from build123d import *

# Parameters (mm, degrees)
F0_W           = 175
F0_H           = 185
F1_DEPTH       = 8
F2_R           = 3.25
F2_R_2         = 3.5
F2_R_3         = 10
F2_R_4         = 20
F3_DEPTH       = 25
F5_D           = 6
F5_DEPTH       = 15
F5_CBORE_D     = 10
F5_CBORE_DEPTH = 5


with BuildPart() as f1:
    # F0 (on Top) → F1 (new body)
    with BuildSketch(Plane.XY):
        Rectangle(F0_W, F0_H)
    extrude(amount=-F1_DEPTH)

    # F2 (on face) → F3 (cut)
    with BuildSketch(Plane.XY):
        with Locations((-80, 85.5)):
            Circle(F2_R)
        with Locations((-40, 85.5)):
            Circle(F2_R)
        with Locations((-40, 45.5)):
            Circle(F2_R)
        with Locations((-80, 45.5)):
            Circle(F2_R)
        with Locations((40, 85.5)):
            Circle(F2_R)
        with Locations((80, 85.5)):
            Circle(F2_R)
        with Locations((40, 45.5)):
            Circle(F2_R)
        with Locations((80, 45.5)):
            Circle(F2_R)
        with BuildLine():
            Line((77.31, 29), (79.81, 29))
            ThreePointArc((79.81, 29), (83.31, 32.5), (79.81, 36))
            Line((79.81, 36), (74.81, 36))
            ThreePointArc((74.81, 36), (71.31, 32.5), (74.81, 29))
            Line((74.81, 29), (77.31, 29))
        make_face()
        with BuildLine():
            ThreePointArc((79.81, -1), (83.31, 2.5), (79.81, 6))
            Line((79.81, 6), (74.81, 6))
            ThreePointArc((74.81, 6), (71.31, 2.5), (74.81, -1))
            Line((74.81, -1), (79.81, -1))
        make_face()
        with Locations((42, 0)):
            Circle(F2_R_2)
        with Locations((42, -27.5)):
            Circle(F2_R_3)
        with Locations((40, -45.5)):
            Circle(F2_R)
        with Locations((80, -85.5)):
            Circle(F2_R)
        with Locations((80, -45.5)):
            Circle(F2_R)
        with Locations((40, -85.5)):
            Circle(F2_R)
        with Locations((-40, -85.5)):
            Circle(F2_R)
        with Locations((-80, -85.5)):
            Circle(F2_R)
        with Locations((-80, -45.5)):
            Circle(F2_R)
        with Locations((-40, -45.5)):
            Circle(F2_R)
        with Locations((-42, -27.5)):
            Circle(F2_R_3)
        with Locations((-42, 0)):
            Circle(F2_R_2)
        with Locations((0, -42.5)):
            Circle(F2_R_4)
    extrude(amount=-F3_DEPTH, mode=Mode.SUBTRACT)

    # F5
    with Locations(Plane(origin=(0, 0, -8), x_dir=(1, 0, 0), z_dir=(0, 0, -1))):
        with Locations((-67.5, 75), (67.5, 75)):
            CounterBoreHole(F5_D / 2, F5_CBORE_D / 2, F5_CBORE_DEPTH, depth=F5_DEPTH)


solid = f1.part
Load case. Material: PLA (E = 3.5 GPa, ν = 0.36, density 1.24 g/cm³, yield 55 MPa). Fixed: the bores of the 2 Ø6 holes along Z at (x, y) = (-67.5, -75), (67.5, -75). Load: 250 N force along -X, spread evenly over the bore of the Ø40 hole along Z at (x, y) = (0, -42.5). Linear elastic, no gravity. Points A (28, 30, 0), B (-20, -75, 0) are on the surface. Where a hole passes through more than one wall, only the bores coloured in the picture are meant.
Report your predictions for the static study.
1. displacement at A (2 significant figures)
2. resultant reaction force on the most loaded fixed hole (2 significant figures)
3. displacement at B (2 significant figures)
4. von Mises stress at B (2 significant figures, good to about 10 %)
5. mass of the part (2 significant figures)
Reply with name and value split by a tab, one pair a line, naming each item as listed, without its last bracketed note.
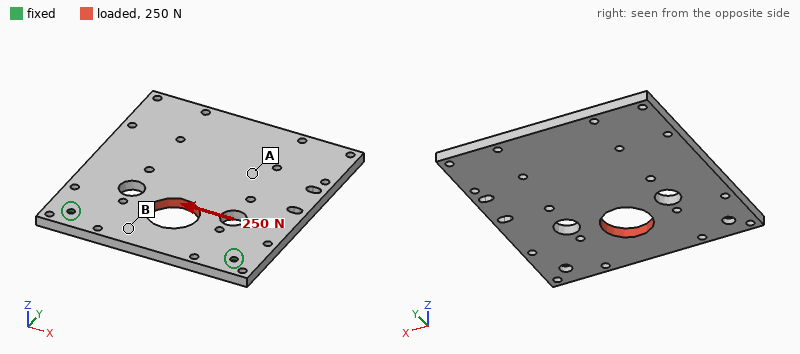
displacement at A	22 µm
resultant reaction force on the most loaded fixed hole	140 N
displacement at B	10 µm
von Mises stress at B	0.32 MPa
mass of the part	290 g
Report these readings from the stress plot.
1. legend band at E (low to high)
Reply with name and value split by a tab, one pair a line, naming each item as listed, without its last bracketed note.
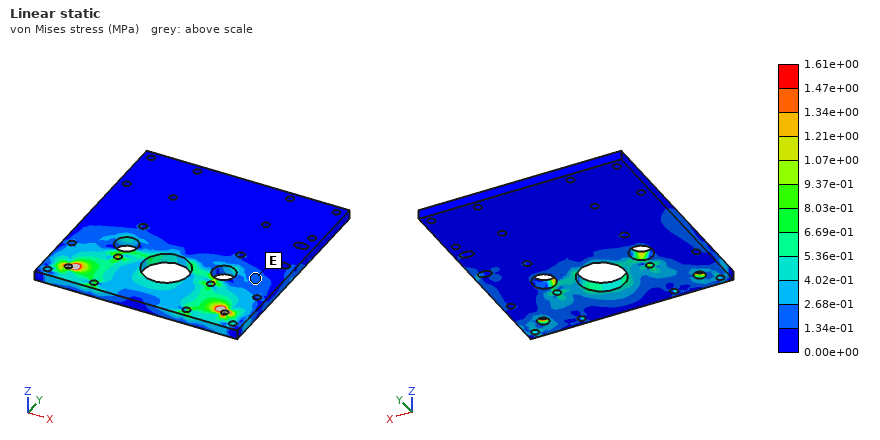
legend band at E	1.34e-01 to 2.68e-01 MPa
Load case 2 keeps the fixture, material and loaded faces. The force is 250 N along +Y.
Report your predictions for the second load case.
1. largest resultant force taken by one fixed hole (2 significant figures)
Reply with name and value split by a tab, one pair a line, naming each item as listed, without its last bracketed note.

largest resultant force taken by one fixed hole	130 N
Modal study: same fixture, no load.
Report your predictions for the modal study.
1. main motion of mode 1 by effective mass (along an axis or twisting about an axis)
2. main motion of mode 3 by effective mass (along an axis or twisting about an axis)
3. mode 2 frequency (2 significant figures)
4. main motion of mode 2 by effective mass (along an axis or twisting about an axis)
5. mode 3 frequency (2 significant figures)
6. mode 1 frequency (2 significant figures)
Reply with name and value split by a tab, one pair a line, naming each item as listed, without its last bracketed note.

main motion of mode 1 by effective mass	along Z
main motion of mode 3 by effective mass	along Z
mode 2 frequency	160 Hz
main motion of mode 2 by effective mass	twisting about Y
mode 3 frequency	360 Hz
mode 1 frequency	45 Hz
